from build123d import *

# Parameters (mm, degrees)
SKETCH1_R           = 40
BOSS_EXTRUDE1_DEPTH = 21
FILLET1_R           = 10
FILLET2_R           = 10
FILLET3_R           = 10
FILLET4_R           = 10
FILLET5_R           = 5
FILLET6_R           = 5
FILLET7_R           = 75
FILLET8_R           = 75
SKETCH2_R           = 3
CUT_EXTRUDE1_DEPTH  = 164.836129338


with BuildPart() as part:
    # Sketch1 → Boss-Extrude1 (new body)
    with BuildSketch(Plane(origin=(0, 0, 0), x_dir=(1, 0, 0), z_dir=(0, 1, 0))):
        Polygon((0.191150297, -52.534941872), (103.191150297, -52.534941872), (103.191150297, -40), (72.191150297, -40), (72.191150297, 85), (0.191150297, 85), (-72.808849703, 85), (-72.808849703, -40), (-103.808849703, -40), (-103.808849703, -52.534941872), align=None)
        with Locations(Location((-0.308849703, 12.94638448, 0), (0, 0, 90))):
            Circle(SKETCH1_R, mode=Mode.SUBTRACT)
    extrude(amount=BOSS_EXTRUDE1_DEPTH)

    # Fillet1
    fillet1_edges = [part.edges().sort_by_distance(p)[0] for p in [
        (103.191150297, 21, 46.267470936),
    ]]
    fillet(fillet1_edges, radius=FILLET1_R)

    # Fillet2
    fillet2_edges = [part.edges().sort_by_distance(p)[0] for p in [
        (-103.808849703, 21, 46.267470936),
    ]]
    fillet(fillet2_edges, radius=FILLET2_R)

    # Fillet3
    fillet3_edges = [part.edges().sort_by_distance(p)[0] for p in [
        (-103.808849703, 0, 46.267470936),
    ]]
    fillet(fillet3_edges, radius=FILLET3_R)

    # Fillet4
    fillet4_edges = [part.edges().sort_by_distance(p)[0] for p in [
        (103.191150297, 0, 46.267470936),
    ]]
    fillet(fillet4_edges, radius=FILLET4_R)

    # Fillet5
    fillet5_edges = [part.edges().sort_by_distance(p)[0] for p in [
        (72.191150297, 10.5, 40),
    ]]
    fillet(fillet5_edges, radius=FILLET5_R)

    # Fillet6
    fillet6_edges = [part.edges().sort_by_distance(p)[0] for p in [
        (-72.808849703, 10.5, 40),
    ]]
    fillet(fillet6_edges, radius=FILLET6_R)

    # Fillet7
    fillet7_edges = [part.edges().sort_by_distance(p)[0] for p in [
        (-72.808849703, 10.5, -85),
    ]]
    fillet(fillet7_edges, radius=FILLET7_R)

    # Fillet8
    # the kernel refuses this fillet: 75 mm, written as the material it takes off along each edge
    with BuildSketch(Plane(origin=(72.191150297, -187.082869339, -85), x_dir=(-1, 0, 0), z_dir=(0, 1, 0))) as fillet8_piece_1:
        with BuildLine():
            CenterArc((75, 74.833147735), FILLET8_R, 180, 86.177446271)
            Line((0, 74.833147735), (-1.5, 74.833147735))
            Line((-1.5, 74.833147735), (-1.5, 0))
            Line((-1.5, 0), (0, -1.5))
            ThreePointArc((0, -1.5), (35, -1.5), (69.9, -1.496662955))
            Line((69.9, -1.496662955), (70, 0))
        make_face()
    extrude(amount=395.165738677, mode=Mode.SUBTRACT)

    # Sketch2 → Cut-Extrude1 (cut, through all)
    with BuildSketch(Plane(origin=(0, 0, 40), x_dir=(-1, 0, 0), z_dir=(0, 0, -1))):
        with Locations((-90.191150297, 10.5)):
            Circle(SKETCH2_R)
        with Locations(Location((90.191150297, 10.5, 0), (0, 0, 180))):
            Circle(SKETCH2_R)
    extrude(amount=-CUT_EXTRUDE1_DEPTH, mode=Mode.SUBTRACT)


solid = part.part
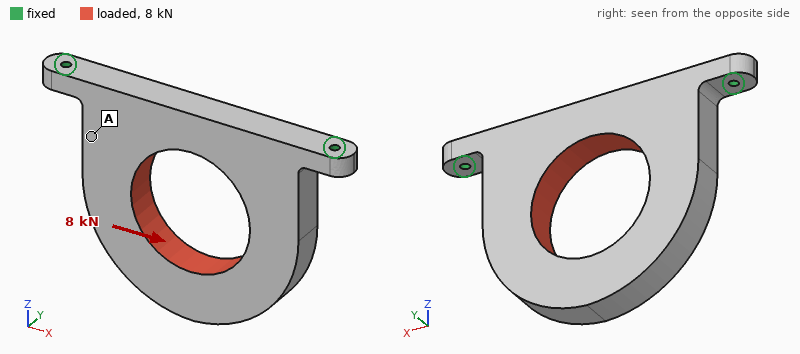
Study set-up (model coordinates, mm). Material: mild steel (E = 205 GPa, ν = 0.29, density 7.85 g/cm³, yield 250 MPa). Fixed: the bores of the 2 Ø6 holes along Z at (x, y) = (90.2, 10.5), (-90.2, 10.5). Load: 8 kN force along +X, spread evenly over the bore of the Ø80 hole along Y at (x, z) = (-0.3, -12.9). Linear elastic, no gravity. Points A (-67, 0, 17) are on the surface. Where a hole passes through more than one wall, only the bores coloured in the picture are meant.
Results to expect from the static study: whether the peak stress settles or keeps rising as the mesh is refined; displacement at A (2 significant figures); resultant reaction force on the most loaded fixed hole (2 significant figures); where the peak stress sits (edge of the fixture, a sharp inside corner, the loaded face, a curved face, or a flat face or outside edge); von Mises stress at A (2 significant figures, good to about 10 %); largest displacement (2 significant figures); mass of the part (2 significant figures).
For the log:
keeps rising
8.2 µm
5.0 kN
edge of the fixture
9.5 MPa
23 µm
2.2 kg
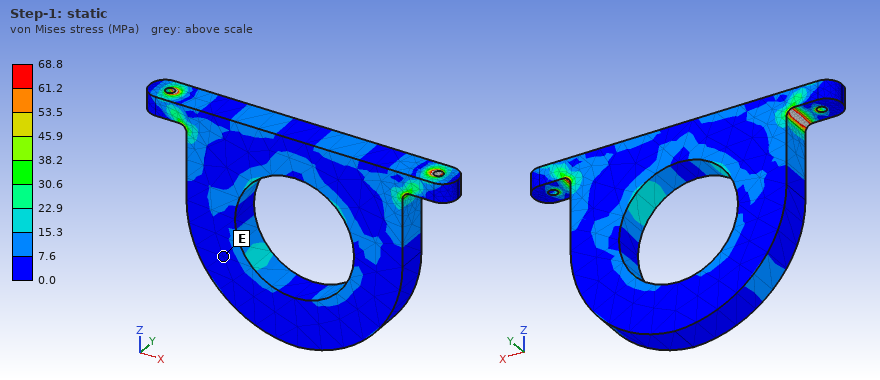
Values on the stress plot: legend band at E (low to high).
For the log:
0.0 to 7.6 MPa
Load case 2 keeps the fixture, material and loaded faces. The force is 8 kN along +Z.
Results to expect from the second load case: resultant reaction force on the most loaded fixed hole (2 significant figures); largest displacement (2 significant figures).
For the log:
4.7 kN
18 µm
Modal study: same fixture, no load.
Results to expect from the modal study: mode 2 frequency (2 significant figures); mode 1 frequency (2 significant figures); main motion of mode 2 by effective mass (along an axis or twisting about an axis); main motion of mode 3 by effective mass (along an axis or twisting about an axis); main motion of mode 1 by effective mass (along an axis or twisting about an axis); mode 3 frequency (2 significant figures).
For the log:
1800 Hz
390 Hz
twisting about Z
along Y
along Y
2200 Hz
